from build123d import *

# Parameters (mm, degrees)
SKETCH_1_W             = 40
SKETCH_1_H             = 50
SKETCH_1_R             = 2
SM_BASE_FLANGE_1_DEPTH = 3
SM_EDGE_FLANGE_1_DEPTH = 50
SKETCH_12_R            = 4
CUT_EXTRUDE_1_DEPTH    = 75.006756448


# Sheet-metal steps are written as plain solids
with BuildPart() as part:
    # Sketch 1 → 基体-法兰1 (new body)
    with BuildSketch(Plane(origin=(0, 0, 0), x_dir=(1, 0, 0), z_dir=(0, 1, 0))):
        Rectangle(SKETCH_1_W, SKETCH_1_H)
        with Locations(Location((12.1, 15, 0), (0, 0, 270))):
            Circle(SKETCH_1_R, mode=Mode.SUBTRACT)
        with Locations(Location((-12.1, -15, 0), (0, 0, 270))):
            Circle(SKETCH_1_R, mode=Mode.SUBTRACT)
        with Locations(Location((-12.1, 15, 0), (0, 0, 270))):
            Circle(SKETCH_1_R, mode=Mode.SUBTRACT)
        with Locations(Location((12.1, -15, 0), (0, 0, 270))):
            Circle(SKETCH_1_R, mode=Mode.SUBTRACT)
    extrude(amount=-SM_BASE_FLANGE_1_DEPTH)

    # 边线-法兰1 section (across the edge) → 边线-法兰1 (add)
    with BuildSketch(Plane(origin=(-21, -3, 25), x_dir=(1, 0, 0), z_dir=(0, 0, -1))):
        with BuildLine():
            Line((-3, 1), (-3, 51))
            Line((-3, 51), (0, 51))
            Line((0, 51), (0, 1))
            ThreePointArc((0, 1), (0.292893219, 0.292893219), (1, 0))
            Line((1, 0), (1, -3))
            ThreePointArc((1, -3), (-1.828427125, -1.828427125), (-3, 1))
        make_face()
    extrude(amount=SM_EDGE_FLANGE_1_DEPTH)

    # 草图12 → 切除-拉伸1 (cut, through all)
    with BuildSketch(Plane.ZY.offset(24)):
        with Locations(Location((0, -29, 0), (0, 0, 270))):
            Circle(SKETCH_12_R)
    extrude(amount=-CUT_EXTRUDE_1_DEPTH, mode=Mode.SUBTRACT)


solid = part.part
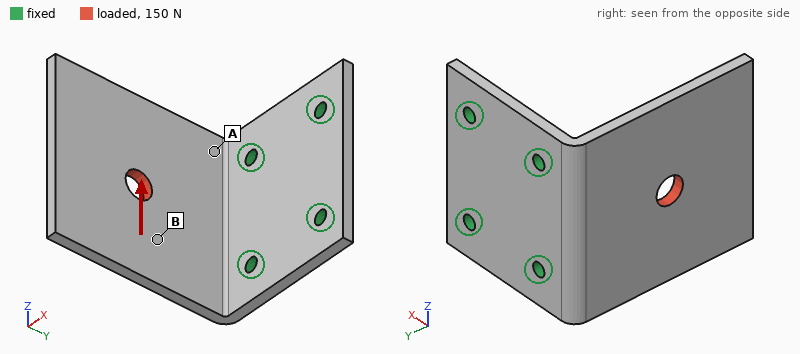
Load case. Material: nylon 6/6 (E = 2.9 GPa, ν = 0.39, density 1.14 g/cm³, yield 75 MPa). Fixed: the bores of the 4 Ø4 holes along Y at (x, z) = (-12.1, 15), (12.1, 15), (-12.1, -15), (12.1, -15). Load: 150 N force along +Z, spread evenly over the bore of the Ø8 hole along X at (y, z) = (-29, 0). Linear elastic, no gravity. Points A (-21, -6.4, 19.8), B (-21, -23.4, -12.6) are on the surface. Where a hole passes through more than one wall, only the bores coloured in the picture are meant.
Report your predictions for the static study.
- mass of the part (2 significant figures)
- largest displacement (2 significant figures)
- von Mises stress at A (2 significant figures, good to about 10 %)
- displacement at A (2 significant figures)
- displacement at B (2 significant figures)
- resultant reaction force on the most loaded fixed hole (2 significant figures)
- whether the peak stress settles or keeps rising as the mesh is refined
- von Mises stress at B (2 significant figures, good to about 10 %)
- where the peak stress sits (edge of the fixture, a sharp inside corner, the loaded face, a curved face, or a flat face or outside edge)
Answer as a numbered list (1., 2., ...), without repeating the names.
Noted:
1. 16 g
2. 1.00 mm
3. 11 MPa
4. 0.28 mm
5. 0.44 mm
6. 160 N
7. keeps rising
8. 3.8 MPa
9. edge of the fixture
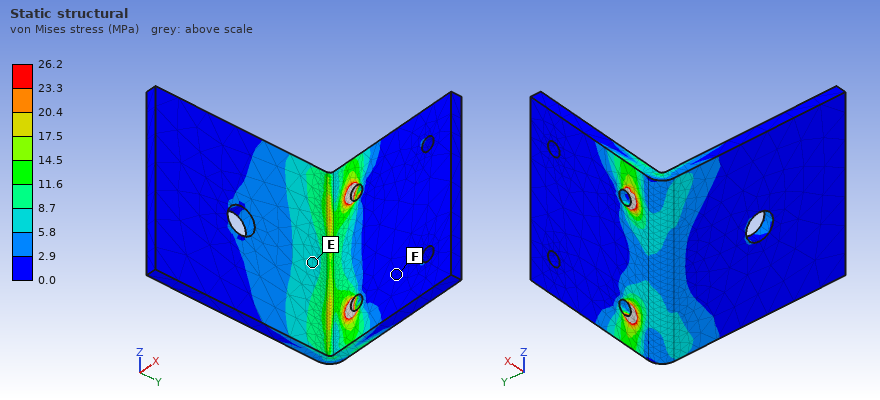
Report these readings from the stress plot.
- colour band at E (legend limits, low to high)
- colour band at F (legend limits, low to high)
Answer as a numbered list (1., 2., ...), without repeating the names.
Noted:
1. 5.8 to 8.7 MPa
2. 0.0 to 2.9 MPa
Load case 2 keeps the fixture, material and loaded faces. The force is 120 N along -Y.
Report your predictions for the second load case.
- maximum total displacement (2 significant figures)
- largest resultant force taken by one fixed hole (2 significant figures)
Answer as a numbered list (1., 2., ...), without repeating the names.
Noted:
1. 1.0 mm
2. 66 N
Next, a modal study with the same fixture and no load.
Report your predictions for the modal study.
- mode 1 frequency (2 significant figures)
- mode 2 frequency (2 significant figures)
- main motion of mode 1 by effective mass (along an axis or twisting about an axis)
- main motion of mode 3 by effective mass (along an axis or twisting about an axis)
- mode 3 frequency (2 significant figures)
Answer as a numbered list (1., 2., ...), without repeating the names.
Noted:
1. 220 Hz
2. 590 Hz
3. along X
4. along Z
5. 930 Hz
